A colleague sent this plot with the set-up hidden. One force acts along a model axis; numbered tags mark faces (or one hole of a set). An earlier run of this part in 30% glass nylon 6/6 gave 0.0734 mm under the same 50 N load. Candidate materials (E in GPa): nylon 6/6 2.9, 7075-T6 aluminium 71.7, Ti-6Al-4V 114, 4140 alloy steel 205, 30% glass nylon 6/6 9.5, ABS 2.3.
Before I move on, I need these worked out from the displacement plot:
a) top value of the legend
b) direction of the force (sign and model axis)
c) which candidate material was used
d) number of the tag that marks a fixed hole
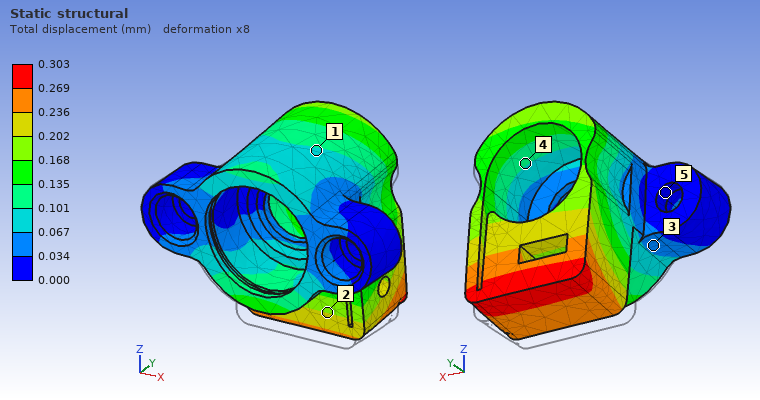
0.303 mm
+Y
ABS
5
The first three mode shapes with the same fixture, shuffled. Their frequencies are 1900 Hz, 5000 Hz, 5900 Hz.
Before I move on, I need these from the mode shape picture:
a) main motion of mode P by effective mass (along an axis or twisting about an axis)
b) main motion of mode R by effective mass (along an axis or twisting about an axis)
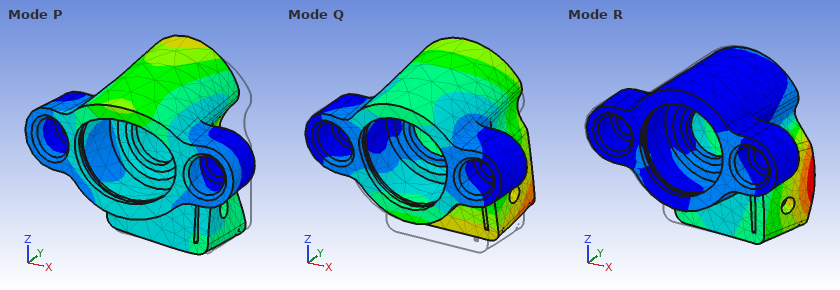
along Y
along X
